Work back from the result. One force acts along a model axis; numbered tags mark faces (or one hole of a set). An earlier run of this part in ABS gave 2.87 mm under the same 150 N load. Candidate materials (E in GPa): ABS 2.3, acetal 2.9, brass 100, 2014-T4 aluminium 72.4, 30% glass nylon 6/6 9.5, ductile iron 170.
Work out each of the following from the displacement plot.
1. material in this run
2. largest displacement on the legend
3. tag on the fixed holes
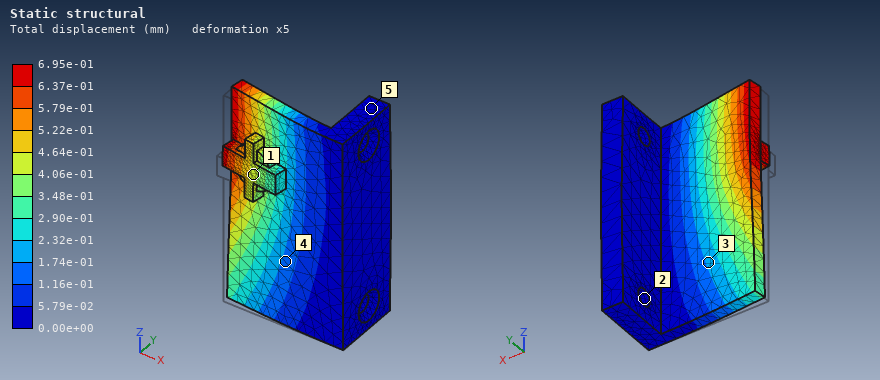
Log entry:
30% glass nylon 6/6
6.95e-01 mm
2
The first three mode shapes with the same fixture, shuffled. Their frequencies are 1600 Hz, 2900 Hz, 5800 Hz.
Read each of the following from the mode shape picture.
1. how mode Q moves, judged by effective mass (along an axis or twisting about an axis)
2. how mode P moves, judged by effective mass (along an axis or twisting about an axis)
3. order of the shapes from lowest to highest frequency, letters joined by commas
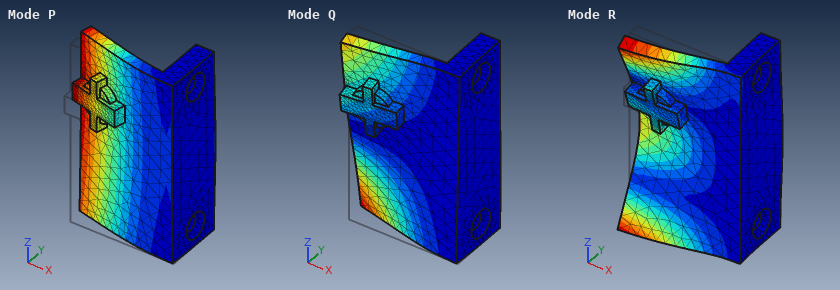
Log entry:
twisting about X
along Y
P, Q, R
